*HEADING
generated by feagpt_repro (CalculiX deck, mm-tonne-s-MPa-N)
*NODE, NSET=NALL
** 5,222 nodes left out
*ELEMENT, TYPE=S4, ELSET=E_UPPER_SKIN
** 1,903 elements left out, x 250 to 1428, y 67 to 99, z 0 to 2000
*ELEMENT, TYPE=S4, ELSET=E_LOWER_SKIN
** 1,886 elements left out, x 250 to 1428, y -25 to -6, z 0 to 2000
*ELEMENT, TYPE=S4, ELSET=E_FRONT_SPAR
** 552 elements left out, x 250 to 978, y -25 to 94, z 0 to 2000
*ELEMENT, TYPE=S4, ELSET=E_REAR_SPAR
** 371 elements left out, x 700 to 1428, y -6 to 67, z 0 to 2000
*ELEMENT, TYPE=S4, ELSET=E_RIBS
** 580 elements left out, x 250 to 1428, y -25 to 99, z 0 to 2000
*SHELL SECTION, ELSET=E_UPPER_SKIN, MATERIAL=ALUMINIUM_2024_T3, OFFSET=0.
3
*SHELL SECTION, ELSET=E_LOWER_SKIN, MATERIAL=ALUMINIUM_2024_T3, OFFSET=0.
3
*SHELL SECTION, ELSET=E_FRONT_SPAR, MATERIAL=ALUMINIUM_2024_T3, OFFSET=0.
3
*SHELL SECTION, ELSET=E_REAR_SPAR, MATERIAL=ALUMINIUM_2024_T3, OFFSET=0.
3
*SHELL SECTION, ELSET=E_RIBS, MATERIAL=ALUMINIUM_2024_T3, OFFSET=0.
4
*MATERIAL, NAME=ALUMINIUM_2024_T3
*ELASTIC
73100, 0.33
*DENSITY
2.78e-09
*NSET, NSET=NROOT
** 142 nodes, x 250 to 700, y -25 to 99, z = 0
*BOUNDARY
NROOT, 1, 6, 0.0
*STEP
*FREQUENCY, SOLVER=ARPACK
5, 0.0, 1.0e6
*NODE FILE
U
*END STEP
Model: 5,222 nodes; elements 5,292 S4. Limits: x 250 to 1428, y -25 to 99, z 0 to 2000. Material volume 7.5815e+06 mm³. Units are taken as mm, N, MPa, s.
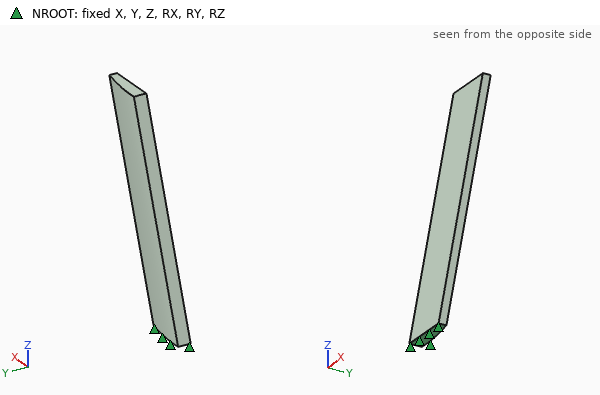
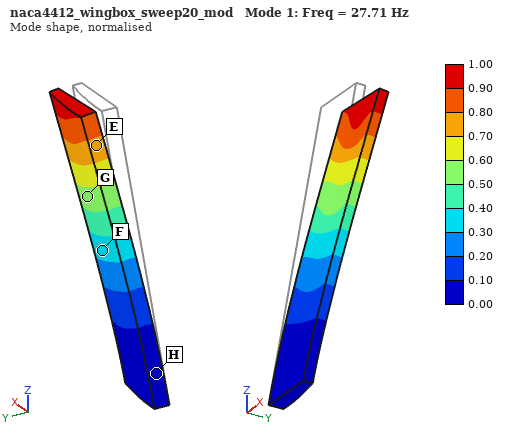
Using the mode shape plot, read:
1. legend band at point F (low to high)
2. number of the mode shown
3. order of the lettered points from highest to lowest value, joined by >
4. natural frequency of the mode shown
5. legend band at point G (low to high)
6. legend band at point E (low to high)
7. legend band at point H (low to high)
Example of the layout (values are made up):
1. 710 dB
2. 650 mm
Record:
1. 0.30 to 0.40
2. 1
3. E > G > F > H
4. 27.71 Hz
5. 0.50 to 0.60
6. 0.70 to 0.80
7. 0.00 to 0.10
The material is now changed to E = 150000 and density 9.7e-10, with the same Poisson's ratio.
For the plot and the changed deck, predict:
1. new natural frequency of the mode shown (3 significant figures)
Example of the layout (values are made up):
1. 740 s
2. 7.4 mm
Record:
1. 67.2 Hz
